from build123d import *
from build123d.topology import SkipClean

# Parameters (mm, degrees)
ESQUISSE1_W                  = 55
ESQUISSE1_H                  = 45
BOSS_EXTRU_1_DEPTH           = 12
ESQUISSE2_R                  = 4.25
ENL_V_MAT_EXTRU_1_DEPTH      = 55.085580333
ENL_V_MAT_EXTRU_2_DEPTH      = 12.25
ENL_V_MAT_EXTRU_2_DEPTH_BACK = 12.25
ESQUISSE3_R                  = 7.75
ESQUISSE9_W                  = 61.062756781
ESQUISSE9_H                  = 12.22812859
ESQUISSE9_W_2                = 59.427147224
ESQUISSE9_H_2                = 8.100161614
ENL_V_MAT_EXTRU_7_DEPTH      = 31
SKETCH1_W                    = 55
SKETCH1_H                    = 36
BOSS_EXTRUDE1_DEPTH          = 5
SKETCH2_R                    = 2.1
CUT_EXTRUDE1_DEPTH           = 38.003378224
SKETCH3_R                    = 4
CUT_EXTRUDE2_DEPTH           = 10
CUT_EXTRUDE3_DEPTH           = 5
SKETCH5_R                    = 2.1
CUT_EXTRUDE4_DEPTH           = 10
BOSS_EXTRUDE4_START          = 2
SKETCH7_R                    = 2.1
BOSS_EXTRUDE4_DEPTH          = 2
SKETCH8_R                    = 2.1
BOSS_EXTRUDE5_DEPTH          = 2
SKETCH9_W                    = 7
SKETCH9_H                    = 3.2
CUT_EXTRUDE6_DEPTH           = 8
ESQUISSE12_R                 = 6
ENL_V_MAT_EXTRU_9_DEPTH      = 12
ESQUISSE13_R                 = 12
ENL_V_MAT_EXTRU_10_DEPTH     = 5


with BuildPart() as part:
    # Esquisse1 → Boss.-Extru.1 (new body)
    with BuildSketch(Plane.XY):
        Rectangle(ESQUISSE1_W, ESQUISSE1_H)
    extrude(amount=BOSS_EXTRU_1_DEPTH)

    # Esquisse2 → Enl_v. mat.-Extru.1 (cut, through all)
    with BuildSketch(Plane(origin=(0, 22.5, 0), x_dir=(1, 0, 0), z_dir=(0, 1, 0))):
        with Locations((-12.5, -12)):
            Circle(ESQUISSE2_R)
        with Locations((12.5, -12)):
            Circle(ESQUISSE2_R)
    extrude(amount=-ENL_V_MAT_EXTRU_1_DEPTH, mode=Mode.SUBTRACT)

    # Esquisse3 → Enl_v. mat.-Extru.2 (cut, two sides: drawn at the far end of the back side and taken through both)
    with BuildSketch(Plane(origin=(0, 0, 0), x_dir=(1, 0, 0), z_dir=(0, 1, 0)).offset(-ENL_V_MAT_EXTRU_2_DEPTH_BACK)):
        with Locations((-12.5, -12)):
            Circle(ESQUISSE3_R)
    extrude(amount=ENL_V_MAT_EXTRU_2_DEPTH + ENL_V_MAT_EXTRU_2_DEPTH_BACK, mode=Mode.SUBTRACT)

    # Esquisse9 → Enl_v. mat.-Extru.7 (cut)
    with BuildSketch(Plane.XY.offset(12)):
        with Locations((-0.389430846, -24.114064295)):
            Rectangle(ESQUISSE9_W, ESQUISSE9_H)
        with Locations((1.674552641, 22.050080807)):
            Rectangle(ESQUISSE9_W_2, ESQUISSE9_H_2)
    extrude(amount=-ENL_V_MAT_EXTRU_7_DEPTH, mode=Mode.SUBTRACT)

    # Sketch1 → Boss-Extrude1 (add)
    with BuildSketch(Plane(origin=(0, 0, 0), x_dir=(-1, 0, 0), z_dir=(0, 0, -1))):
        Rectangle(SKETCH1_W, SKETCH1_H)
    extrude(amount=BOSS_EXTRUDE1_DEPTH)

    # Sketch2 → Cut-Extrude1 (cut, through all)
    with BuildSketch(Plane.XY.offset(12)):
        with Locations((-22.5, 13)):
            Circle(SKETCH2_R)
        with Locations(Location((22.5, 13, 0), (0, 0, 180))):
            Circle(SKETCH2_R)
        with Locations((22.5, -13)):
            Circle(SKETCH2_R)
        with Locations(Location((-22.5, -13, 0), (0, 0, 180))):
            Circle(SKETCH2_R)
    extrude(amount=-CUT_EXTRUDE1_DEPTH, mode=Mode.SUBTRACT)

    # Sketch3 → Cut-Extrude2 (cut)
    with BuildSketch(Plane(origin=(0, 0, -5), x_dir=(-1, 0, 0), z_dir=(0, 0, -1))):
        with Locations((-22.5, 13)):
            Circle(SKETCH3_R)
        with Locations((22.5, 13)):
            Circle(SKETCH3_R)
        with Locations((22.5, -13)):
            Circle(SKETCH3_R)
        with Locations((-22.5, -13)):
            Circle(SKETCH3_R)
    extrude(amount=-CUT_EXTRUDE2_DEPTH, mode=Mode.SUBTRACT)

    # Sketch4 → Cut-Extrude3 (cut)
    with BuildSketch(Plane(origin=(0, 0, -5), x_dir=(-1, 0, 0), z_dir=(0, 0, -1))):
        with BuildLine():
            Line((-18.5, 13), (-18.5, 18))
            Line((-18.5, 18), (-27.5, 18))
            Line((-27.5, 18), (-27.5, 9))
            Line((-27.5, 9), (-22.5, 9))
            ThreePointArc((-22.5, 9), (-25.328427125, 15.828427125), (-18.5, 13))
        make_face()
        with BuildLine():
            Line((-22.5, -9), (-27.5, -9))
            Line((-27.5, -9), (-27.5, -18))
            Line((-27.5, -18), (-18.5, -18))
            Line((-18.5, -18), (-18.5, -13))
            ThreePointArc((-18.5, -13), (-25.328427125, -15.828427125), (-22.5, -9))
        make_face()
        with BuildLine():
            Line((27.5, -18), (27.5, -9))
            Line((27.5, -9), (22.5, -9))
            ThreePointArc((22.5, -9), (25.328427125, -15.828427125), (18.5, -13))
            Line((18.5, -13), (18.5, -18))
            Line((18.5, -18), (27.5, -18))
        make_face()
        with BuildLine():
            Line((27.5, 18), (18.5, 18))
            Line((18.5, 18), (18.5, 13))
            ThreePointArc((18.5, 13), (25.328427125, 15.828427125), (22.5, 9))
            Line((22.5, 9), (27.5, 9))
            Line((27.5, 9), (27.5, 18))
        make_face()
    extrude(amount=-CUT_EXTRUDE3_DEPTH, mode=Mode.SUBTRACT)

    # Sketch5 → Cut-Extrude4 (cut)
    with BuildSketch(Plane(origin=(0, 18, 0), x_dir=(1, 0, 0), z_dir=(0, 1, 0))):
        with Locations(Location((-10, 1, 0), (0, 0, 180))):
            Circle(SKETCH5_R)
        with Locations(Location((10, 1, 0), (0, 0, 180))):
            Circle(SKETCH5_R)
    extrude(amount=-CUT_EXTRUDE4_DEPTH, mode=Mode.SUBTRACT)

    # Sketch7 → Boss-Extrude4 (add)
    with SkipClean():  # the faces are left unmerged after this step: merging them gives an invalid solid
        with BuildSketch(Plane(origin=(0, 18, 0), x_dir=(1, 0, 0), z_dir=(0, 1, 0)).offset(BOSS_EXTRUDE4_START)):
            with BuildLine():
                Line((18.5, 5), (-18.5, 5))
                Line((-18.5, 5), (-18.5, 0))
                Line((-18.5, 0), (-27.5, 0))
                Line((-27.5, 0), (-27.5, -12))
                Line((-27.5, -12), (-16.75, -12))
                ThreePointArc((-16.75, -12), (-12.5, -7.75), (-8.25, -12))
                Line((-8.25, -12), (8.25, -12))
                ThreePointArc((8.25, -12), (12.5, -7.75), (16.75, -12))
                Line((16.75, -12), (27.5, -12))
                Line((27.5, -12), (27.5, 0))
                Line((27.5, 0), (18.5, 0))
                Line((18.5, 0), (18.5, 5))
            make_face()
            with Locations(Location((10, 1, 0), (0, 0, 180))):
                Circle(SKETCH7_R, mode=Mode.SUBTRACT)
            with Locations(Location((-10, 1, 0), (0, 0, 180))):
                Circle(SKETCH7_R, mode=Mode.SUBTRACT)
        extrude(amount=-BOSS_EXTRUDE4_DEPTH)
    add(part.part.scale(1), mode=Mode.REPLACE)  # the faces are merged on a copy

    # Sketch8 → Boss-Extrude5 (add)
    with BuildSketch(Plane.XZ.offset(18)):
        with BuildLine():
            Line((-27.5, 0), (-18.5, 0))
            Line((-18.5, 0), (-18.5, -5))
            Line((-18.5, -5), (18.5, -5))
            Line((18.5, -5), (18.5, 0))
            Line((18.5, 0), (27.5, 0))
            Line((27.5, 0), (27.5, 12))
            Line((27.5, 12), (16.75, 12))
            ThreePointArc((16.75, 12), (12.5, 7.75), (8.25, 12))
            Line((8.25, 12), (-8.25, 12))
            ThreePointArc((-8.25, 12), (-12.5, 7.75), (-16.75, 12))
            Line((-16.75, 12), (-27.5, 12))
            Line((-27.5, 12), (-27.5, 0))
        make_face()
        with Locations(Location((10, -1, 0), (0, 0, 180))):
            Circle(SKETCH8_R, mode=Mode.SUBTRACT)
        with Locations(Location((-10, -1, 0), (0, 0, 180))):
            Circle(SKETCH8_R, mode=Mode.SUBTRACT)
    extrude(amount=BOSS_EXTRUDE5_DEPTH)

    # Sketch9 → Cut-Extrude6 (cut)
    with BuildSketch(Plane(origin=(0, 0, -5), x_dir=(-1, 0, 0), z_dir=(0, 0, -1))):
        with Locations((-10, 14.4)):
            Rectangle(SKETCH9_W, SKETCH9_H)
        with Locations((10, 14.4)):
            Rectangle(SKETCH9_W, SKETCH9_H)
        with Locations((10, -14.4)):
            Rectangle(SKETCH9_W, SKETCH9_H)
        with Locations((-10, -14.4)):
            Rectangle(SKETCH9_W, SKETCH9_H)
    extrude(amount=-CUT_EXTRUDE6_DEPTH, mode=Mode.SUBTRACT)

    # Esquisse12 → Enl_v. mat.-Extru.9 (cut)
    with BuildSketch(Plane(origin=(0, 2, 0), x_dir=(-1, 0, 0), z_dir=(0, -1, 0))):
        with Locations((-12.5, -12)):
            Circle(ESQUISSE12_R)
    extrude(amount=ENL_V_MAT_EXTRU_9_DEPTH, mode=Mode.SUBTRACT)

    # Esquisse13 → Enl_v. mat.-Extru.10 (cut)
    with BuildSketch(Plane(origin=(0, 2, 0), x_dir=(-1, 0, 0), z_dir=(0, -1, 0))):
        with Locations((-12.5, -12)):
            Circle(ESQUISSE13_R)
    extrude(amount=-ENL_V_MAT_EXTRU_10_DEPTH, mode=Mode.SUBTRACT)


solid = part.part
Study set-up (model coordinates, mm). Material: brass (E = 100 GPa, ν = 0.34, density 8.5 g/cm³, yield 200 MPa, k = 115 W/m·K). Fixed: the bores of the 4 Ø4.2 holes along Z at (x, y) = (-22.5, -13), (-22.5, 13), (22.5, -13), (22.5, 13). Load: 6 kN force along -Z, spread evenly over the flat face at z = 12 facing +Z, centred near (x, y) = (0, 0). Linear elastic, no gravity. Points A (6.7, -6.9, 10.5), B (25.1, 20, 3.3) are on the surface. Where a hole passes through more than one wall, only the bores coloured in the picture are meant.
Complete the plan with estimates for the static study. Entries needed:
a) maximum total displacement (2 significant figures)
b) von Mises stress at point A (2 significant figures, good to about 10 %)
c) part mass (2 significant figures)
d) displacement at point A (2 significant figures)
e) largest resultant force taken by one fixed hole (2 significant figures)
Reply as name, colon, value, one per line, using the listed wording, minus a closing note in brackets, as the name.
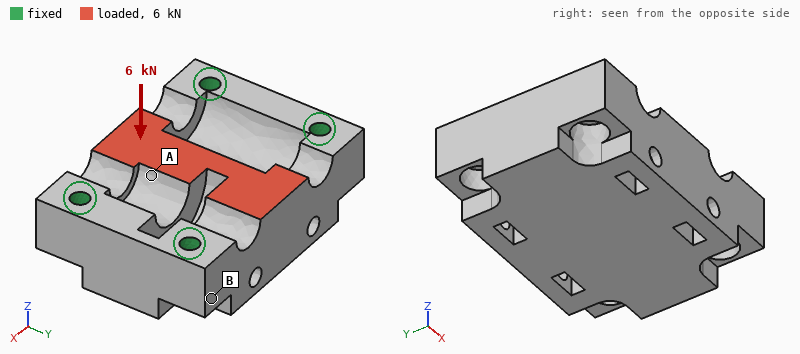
maximum total displacement: 12 µm
von Mises stress at point A: 15 MPa
part mass: 240 g
displacement at point A: 8.9 µm
largest resultant force taken by one fixed hole: 2.0 kN
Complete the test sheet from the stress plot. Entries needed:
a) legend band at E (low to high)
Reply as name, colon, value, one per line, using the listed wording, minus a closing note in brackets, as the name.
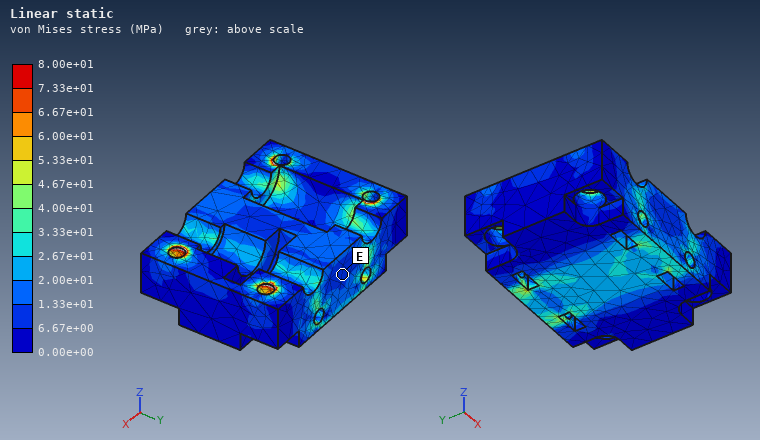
legend band at E: 6.67e+00 to 1.33e+01 MPa
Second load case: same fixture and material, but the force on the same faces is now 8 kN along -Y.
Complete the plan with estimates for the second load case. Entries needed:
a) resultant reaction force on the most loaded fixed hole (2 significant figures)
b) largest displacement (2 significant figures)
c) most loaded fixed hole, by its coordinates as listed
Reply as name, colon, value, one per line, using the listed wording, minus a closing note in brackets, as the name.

resultant reaction force on the most loaded fixed hole: 2.4 kN
largest displacement: 29 µm
most loaded fixed hole, by its coordinates as listed: (22.5, -13)
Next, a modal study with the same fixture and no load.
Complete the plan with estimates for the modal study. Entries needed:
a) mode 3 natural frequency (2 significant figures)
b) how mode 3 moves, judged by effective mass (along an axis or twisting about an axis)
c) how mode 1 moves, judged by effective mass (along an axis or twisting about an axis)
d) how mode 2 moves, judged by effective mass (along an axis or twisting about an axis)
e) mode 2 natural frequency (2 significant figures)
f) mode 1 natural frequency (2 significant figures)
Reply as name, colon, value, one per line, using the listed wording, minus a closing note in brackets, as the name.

mode 3 natural frequency: 13 kHz
how mode 3 moves, judged by effective mass: along Y
how mode 1 moves, judged by effective mass: along Z
how mode 2 moves, judged by effective mass: along Y
mode 2 natural frequency: 12 kHz
mode 1 natural frequency: 12 kHz
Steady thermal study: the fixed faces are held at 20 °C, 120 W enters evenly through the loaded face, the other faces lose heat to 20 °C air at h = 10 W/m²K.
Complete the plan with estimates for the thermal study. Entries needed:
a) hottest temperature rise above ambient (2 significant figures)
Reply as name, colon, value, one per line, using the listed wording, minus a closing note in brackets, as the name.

hottest temperature rise above ambient: 45 K
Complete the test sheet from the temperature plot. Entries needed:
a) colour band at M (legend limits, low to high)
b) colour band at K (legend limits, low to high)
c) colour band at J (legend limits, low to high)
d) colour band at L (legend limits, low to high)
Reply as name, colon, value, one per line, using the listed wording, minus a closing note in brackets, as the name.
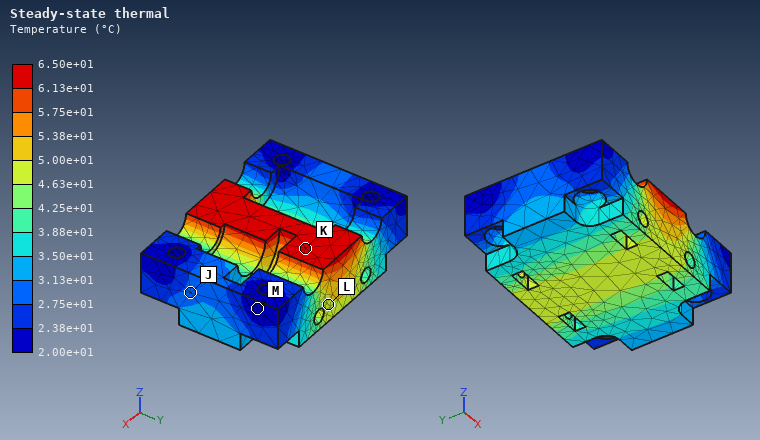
colour band at M: 2.00e+01 to 2.38e+01 °C
colour band at K: 6.13e+01 to 6.50e+01 °C
colour band at J: 2.75e+01 to 3.13e+01 °C
colour band at L: 4.63e+01 to 5.00e+01 °C
